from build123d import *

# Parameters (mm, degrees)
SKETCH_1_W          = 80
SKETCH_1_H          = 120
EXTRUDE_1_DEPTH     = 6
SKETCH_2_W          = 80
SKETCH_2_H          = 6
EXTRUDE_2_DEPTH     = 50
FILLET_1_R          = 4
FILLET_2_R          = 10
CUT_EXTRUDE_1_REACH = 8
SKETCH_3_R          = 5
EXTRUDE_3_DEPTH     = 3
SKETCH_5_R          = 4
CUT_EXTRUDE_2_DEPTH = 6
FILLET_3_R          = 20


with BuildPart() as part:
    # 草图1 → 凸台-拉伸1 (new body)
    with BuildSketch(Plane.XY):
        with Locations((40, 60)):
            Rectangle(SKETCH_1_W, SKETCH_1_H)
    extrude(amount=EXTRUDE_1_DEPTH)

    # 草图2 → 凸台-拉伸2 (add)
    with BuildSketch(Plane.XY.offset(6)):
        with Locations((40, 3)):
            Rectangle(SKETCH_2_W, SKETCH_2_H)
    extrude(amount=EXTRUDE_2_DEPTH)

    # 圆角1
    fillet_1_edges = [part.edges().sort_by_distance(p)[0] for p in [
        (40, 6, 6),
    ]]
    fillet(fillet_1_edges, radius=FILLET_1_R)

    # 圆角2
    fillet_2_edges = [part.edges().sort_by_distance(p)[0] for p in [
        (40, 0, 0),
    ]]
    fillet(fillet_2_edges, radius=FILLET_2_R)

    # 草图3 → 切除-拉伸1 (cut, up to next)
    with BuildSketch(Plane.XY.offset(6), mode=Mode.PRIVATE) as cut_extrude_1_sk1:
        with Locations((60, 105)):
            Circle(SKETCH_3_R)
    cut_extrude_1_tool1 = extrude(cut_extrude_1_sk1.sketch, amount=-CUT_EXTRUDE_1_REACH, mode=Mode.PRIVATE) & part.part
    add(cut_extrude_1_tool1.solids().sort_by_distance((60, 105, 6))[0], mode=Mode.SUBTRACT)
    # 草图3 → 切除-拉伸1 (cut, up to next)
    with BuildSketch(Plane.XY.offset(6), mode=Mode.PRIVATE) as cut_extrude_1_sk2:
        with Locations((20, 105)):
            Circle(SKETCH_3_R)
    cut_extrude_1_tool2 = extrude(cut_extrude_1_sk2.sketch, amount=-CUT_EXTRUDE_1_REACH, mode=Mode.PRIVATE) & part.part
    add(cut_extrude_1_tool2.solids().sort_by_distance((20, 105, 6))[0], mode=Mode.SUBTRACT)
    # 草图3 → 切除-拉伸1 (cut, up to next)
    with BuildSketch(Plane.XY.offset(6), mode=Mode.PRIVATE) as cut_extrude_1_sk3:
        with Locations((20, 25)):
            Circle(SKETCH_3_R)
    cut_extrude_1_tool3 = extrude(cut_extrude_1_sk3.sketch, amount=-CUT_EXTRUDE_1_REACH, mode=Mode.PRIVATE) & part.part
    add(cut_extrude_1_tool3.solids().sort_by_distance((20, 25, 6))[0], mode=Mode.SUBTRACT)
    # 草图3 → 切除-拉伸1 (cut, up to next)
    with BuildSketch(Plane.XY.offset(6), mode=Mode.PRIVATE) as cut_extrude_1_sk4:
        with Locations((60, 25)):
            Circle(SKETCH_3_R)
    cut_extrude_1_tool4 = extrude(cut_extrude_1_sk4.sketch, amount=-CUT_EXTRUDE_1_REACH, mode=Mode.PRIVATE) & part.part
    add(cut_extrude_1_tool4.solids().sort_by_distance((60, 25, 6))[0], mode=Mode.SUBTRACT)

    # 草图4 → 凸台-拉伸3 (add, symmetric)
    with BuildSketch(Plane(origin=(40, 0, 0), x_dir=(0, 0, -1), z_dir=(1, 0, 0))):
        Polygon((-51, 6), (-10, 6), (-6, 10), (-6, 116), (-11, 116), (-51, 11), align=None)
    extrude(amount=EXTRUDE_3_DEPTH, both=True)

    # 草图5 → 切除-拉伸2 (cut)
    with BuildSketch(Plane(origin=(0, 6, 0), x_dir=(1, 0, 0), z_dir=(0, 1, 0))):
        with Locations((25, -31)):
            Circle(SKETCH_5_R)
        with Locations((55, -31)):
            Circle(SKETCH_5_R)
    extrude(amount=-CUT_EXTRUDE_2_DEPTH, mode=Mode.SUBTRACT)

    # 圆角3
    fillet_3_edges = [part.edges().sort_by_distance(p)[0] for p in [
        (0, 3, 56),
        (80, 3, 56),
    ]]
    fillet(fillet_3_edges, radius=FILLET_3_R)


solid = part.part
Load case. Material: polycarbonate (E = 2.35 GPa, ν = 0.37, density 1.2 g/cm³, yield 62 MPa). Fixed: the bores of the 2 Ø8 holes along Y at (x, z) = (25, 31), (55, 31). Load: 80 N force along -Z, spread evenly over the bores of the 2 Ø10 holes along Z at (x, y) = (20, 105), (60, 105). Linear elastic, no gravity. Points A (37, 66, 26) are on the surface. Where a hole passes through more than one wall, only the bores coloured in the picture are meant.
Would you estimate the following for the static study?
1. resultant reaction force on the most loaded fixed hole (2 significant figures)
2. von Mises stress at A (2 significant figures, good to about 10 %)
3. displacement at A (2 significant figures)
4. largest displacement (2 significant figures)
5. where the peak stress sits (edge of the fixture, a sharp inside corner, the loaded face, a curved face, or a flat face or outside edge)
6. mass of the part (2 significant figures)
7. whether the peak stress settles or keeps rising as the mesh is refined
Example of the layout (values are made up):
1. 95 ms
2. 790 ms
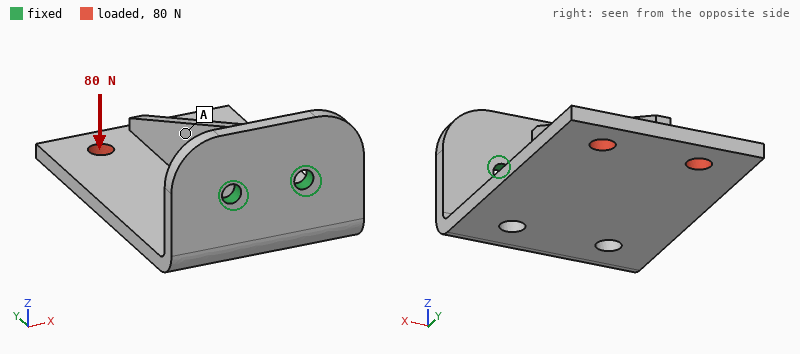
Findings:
1. 42 N
2. 2.0 MPa
3. 0.75 mm
4. 1.7 mm
5. edge of the fixture
6. 110 g
7. keeps rising
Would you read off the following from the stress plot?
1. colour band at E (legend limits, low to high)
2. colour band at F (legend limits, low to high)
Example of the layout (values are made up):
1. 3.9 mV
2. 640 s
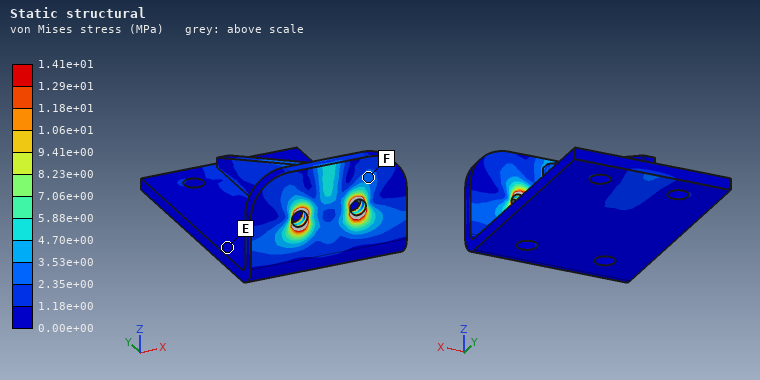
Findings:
1. 0.00e+00 to 1.18e+00 MPa
2. 2.35e+00 to 3.53e+00 MPa
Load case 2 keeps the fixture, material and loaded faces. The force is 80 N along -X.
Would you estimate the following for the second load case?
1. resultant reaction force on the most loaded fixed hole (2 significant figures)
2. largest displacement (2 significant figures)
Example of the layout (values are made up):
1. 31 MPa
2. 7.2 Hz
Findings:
1. 240 N
2. 1.6 mm
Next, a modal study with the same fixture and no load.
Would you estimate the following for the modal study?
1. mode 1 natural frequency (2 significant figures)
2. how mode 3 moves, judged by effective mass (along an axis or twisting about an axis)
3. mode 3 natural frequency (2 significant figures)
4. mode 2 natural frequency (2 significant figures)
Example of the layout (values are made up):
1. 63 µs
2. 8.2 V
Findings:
1. 200 Hz
2. twisting about Y
3. 360 Hz
4. 200 Hz
